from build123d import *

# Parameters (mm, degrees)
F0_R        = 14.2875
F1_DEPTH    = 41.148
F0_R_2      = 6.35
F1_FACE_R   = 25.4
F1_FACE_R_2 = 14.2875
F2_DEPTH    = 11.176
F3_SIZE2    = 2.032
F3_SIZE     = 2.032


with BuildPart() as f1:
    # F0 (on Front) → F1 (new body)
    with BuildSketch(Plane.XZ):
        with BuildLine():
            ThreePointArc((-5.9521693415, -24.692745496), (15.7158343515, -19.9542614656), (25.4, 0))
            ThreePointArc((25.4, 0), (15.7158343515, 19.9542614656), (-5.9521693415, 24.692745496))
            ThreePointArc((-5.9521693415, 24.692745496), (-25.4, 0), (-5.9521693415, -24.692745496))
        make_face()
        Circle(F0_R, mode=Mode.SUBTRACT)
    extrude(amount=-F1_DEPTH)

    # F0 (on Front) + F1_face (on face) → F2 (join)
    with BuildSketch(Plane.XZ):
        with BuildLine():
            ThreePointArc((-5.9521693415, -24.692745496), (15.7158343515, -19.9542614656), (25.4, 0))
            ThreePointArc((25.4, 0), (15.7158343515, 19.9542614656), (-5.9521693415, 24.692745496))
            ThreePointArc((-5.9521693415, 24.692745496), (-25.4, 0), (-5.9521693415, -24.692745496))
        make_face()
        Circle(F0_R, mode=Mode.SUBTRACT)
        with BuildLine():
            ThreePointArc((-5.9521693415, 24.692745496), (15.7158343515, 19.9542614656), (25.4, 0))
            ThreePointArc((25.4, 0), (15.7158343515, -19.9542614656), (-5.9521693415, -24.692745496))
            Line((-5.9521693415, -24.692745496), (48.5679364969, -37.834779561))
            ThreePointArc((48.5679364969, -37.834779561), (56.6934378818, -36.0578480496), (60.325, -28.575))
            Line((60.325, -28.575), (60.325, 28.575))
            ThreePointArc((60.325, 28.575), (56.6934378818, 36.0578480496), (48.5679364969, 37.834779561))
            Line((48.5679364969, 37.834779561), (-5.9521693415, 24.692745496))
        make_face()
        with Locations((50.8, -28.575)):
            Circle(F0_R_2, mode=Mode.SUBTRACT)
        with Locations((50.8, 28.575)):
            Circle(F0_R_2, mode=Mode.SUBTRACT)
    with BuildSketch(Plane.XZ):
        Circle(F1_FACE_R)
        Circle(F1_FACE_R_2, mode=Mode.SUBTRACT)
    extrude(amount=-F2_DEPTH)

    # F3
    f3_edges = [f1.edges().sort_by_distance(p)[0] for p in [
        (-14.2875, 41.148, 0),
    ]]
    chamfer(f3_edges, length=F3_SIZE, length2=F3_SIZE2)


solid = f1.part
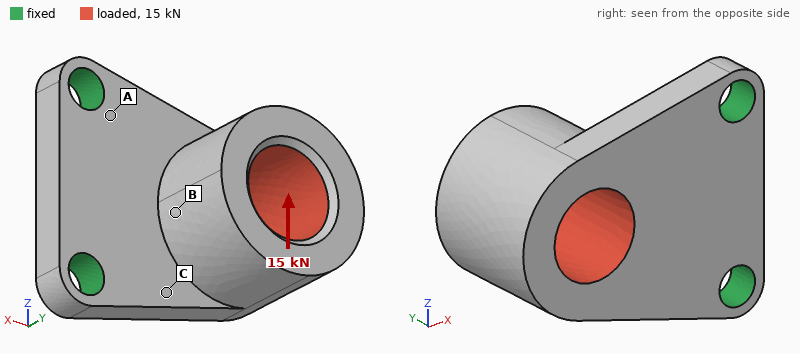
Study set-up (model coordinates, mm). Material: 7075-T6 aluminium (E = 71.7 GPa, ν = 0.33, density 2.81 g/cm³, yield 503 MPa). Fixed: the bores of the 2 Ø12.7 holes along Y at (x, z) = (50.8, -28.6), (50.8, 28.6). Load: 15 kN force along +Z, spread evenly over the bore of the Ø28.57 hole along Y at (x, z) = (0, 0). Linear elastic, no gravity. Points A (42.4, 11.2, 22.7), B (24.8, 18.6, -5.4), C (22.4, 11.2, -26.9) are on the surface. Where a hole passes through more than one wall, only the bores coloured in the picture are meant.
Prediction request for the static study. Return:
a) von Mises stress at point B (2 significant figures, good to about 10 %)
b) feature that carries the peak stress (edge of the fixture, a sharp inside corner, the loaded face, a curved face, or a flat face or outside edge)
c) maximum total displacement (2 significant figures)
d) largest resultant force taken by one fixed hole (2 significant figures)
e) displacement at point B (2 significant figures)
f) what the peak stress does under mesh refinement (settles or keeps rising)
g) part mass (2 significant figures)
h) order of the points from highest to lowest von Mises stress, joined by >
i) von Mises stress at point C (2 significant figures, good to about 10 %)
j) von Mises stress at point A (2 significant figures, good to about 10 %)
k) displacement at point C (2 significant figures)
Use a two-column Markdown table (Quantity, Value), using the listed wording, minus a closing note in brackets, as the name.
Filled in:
| Quantity | Value |
|---|---|
| von Mises stress at point B | 27 MPa |
| feature that carries the peak stress | edge of the fixture |
| maximum total displacement | 0.23 mm |
| largest resultant force taken by one fixed hole | 15 kN |
| displacement at point B | 0.076 mm |
| what the peak stress does under mesh refinement | keeps rising |
| part mass | 240 g |
| order of the points from highest to lowest von Mises stress, joined by > | C > A > B |
| von Mises stress at point C | 100 MPa |
| von Mises stress at point A | 59 MPa |
| displacement at point C | 0.068 mm |
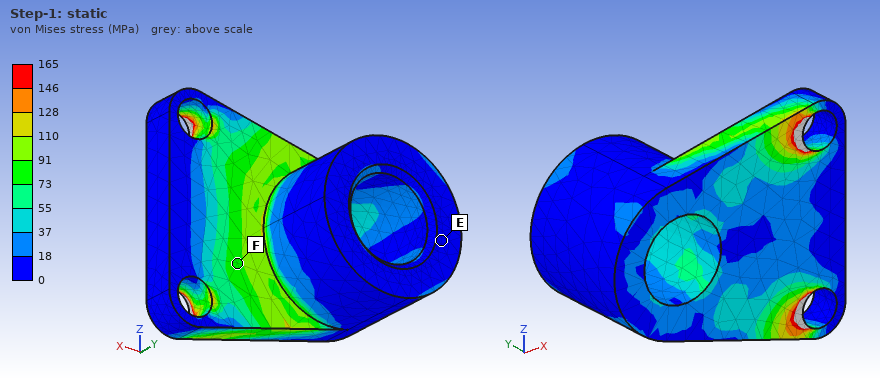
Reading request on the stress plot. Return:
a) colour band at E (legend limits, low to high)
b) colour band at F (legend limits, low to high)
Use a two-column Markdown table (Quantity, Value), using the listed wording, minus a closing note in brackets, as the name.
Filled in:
| Quantity | Value |
|---|---|
| colour band at E | 0 to 18 MPa |
| colour band at F | 73 to 91 MPa |
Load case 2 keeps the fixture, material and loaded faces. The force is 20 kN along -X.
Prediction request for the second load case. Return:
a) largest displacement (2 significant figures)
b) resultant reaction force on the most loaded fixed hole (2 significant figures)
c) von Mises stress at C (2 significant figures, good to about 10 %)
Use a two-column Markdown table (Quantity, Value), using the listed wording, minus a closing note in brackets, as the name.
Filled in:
| Quantity | Value |
|---|---|
| largest displacement | 1.2 mm |
| resultant reaction force on the most loaded fixed hole | 11 kN |
| von Mises stress at C | 190 MPa |
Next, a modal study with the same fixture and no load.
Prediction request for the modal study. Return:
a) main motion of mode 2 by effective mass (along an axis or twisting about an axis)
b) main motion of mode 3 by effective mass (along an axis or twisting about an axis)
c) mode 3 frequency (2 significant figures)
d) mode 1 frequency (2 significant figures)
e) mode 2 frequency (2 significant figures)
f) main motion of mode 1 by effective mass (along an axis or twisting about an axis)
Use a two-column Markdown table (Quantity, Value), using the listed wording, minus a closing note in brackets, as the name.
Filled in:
| Quantity | Value |
|---|---|
| main motion of mode 2 by effective mass | along Z |
| main motion of mode 3 by effective mass | along Z |
| mode 3 frequency | 6100 Hz |
| mode 1 frequency | 1200 Hz |
| mode 2 frequency | 3500 Hz |
| main motion of mode 1 by effective mass | along Y |
